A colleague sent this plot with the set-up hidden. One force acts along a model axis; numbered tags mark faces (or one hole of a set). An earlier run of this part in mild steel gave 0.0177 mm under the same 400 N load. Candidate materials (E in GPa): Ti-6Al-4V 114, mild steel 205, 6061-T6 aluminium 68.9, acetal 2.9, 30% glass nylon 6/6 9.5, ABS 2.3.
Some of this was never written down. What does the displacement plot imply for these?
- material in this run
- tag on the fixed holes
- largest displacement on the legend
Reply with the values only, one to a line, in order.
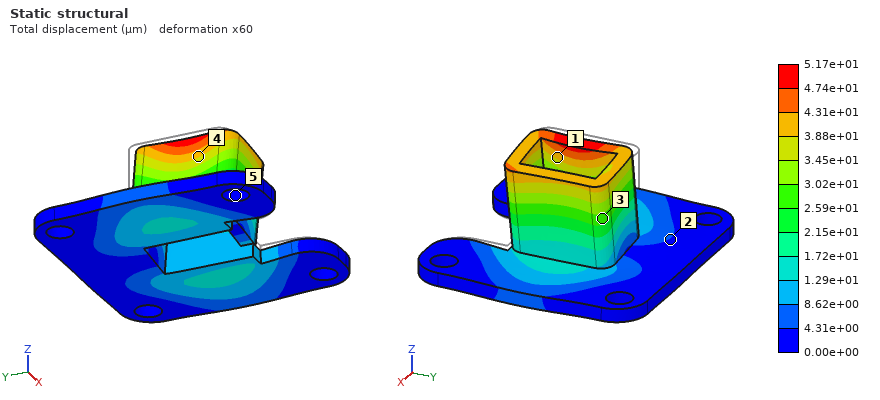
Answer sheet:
6061-T6 aluminium
5
5.17e+01 µm
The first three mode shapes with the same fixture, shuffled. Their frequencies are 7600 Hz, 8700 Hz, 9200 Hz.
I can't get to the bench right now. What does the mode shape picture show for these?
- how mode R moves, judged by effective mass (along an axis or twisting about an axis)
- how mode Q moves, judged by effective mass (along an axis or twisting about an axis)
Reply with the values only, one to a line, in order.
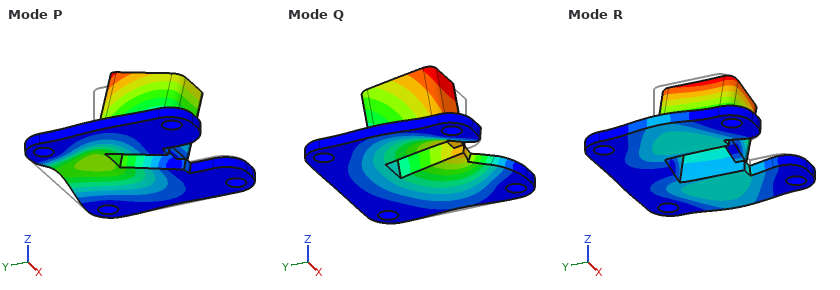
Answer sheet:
along X
along Z
